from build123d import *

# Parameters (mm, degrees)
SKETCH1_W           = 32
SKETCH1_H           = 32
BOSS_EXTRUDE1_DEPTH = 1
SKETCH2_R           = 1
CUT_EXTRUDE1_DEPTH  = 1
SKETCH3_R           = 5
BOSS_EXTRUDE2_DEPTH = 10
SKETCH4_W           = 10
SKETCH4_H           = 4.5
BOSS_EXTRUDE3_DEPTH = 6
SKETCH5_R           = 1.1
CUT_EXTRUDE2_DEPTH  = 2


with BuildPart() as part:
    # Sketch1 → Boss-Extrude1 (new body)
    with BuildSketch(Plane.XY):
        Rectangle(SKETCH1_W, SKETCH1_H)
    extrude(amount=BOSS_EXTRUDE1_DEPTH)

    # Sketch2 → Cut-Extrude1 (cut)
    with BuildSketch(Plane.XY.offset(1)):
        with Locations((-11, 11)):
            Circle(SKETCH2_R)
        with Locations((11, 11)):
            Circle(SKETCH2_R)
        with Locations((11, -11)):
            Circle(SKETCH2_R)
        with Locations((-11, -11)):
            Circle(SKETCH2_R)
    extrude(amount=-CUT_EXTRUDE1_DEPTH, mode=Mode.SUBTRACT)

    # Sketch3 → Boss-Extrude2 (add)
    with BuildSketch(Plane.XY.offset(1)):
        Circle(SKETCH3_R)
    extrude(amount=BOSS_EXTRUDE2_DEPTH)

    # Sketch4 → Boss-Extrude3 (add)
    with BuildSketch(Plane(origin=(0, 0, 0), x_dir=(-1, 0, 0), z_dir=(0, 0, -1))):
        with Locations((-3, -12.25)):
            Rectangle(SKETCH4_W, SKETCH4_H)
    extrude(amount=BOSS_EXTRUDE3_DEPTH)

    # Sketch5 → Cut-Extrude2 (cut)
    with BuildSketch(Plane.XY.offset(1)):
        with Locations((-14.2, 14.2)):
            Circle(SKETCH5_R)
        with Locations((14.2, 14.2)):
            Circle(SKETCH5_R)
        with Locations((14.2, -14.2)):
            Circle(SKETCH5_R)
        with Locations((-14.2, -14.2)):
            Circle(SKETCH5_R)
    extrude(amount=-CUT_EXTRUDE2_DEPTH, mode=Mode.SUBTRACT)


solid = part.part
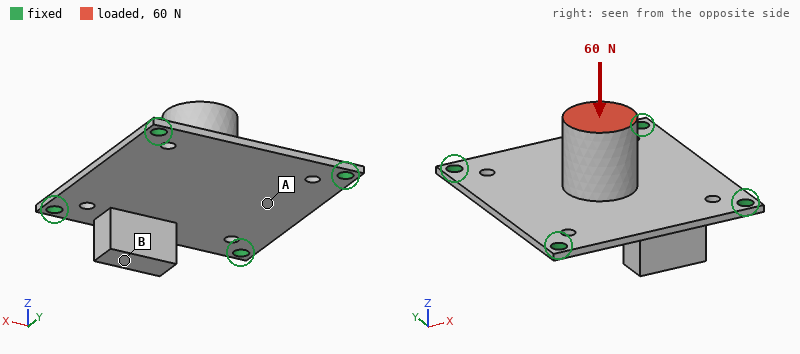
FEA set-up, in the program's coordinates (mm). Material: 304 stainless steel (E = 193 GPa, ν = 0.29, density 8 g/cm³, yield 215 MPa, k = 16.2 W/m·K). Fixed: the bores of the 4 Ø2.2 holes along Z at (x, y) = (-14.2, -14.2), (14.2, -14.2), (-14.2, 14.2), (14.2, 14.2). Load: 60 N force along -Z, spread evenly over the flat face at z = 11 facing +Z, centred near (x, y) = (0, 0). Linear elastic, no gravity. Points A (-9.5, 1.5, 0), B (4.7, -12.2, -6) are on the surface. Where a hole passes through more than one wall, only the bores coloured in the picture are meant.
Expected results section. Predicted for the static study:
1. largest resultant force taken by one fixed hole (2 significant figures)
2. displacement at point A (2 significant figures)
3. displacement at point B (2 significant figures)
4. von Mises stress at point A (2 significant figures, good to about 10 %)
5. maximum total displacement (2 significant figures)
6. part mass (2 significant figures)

16 N
17 µm
13 µm
23 MPa
22 µm
16 g
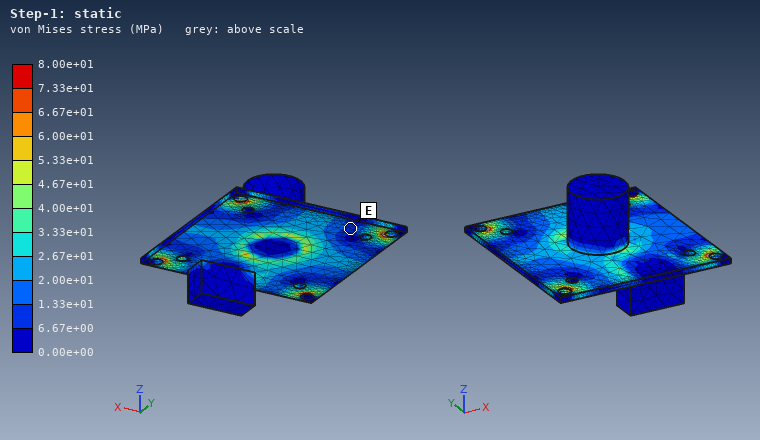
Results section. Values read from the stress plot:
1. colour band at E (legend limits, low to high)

6.67e+00 to 1.33e+01 MPa
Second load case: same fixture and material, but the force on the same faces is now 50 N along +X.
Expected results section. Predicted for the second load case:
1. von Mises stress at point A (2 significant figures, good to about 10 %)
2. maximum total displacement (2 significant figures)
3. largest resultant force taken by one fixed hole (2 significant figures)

22 MPa
21 µm
19 N
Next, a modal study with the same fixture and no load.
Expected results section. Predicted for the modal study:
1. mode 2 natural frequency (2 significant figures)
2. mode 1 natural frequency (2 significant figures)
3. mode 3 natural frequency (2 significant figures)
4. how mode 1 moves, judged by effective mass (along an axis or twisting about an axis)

4200 Hz
2700 Hz
4600 Hz
along Z
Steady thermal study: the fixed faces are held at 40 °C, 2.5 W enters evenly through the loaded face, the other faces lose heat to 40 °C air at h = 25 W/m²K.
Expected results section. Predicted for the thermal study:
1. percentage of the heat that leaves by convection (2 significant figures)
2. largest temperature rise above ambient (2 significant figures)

52 %
55 K
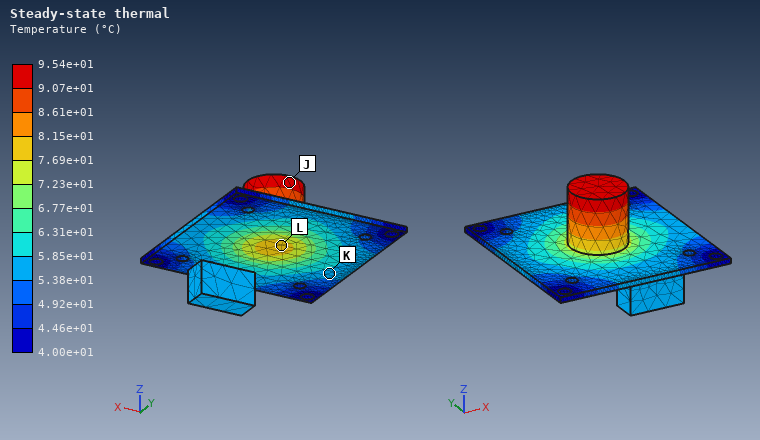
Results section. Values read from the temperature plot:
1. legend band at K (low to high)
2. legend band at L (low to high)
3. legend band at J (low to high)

5.38e+01 to 5.85e+01 °C
7.69e+01 to 8.15e+01 °C
9.07e+01 to 9.54e+01 °C
